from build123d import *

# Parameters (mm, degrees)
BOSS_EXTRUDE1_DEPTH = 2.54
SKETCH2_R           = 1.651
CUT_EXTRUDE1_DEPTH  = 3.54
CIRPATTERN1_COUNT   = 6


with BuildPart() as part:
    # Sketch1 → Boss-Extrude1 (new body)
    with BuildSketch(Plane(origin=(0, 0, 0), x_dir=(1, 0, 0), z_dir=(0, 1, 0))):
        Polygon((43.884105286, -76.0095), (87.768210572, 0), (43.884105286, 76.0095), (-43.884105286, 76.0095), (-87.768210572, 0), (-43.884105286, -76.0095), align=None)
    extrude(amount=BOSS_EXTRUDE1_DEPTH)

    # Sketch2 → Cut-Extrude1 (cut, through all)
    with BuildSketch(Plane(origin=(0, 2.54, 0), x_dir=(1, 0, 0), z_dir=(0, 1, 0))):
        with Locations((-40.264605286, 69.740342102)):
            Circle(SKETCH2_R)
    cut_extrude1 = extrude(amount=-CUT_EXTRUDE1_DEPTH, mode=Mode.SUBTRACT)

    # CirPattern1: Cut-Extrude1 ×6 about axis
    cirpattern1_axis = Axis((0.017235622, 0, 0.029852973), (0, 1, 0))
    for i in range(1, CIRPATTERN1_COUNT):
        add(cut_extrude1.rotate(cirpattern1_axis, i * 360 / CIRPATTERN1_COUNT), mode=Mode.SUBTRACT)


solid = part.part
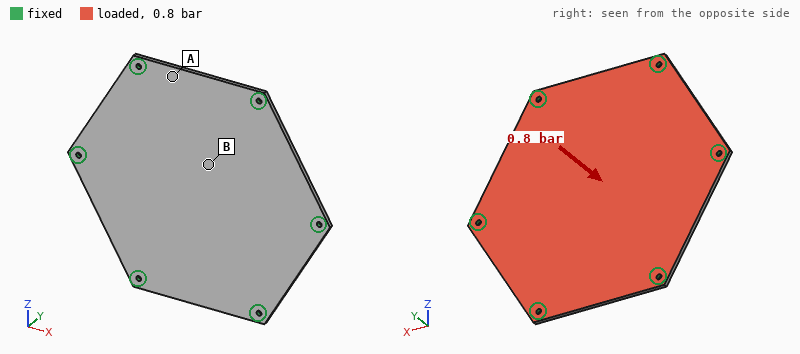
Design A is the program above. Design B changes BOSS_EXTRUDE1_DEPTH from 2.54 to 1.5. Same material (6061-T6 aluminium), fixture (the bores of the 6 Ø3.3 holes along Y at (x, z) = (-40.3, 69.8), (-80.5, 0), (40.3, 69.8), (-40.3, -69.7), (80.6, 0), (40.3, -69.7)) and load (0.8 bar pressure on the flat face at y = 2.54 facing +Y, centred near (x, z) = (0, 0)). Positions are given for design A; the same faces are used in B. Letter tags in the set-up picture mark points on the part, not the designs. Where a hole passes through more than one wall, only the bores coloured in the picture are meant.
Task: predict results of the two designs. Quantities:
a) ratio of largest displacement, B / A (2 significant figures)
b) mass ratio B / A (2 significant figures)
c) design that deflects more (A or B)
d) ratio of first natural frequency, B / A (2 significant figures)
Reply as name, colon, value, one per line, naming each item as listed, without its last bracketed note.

ratio of largest displacement, B / A: 4.7
mass ratio B / A: 0.59
design that deflects more: B
ratio of first natural frequency, B / A: 0.60
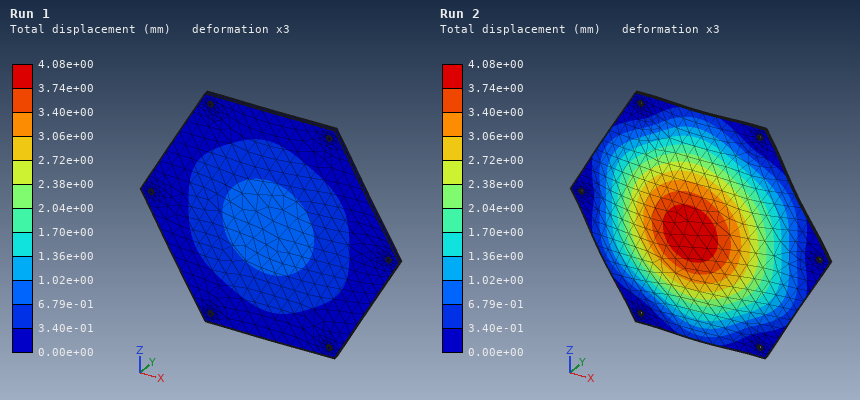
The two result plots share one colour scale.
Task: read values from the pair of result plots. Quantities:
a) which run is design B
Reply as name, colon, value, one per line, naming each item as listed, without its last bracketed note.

which run is design B: Run 2
